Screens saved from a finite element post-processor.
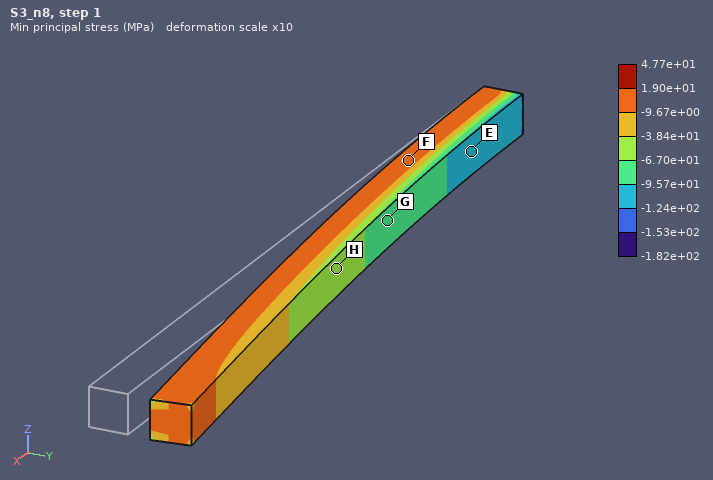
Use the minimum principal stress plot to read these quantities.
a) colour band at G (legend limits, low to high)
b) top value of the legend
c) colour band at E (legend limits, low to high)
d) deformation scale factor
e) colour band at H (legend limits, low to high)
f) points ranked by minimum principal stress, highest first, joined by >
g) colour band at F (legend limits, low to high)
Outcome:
-9.57e+01 to -6.70e+01 MPa
4.77e+01 MPa
-1.24e+02 to -9.57e+01 MPa
10
-6.70e+01 to -3.84e+01 MPa
F > H > G > E
-9.67e+00 to 1.90e+01 MPa
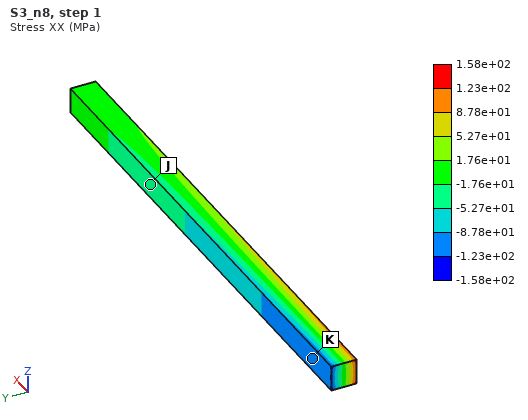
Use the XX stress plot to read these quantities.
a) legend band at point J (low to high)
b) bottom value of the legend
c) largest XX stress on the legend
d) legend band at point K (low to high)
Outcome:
-5.27e+01 to -1.76e+01 MPa
-1.58e+02 MPa
1.58e+02 MPa
-1.23e+02 to -8.78e+01 MPa
